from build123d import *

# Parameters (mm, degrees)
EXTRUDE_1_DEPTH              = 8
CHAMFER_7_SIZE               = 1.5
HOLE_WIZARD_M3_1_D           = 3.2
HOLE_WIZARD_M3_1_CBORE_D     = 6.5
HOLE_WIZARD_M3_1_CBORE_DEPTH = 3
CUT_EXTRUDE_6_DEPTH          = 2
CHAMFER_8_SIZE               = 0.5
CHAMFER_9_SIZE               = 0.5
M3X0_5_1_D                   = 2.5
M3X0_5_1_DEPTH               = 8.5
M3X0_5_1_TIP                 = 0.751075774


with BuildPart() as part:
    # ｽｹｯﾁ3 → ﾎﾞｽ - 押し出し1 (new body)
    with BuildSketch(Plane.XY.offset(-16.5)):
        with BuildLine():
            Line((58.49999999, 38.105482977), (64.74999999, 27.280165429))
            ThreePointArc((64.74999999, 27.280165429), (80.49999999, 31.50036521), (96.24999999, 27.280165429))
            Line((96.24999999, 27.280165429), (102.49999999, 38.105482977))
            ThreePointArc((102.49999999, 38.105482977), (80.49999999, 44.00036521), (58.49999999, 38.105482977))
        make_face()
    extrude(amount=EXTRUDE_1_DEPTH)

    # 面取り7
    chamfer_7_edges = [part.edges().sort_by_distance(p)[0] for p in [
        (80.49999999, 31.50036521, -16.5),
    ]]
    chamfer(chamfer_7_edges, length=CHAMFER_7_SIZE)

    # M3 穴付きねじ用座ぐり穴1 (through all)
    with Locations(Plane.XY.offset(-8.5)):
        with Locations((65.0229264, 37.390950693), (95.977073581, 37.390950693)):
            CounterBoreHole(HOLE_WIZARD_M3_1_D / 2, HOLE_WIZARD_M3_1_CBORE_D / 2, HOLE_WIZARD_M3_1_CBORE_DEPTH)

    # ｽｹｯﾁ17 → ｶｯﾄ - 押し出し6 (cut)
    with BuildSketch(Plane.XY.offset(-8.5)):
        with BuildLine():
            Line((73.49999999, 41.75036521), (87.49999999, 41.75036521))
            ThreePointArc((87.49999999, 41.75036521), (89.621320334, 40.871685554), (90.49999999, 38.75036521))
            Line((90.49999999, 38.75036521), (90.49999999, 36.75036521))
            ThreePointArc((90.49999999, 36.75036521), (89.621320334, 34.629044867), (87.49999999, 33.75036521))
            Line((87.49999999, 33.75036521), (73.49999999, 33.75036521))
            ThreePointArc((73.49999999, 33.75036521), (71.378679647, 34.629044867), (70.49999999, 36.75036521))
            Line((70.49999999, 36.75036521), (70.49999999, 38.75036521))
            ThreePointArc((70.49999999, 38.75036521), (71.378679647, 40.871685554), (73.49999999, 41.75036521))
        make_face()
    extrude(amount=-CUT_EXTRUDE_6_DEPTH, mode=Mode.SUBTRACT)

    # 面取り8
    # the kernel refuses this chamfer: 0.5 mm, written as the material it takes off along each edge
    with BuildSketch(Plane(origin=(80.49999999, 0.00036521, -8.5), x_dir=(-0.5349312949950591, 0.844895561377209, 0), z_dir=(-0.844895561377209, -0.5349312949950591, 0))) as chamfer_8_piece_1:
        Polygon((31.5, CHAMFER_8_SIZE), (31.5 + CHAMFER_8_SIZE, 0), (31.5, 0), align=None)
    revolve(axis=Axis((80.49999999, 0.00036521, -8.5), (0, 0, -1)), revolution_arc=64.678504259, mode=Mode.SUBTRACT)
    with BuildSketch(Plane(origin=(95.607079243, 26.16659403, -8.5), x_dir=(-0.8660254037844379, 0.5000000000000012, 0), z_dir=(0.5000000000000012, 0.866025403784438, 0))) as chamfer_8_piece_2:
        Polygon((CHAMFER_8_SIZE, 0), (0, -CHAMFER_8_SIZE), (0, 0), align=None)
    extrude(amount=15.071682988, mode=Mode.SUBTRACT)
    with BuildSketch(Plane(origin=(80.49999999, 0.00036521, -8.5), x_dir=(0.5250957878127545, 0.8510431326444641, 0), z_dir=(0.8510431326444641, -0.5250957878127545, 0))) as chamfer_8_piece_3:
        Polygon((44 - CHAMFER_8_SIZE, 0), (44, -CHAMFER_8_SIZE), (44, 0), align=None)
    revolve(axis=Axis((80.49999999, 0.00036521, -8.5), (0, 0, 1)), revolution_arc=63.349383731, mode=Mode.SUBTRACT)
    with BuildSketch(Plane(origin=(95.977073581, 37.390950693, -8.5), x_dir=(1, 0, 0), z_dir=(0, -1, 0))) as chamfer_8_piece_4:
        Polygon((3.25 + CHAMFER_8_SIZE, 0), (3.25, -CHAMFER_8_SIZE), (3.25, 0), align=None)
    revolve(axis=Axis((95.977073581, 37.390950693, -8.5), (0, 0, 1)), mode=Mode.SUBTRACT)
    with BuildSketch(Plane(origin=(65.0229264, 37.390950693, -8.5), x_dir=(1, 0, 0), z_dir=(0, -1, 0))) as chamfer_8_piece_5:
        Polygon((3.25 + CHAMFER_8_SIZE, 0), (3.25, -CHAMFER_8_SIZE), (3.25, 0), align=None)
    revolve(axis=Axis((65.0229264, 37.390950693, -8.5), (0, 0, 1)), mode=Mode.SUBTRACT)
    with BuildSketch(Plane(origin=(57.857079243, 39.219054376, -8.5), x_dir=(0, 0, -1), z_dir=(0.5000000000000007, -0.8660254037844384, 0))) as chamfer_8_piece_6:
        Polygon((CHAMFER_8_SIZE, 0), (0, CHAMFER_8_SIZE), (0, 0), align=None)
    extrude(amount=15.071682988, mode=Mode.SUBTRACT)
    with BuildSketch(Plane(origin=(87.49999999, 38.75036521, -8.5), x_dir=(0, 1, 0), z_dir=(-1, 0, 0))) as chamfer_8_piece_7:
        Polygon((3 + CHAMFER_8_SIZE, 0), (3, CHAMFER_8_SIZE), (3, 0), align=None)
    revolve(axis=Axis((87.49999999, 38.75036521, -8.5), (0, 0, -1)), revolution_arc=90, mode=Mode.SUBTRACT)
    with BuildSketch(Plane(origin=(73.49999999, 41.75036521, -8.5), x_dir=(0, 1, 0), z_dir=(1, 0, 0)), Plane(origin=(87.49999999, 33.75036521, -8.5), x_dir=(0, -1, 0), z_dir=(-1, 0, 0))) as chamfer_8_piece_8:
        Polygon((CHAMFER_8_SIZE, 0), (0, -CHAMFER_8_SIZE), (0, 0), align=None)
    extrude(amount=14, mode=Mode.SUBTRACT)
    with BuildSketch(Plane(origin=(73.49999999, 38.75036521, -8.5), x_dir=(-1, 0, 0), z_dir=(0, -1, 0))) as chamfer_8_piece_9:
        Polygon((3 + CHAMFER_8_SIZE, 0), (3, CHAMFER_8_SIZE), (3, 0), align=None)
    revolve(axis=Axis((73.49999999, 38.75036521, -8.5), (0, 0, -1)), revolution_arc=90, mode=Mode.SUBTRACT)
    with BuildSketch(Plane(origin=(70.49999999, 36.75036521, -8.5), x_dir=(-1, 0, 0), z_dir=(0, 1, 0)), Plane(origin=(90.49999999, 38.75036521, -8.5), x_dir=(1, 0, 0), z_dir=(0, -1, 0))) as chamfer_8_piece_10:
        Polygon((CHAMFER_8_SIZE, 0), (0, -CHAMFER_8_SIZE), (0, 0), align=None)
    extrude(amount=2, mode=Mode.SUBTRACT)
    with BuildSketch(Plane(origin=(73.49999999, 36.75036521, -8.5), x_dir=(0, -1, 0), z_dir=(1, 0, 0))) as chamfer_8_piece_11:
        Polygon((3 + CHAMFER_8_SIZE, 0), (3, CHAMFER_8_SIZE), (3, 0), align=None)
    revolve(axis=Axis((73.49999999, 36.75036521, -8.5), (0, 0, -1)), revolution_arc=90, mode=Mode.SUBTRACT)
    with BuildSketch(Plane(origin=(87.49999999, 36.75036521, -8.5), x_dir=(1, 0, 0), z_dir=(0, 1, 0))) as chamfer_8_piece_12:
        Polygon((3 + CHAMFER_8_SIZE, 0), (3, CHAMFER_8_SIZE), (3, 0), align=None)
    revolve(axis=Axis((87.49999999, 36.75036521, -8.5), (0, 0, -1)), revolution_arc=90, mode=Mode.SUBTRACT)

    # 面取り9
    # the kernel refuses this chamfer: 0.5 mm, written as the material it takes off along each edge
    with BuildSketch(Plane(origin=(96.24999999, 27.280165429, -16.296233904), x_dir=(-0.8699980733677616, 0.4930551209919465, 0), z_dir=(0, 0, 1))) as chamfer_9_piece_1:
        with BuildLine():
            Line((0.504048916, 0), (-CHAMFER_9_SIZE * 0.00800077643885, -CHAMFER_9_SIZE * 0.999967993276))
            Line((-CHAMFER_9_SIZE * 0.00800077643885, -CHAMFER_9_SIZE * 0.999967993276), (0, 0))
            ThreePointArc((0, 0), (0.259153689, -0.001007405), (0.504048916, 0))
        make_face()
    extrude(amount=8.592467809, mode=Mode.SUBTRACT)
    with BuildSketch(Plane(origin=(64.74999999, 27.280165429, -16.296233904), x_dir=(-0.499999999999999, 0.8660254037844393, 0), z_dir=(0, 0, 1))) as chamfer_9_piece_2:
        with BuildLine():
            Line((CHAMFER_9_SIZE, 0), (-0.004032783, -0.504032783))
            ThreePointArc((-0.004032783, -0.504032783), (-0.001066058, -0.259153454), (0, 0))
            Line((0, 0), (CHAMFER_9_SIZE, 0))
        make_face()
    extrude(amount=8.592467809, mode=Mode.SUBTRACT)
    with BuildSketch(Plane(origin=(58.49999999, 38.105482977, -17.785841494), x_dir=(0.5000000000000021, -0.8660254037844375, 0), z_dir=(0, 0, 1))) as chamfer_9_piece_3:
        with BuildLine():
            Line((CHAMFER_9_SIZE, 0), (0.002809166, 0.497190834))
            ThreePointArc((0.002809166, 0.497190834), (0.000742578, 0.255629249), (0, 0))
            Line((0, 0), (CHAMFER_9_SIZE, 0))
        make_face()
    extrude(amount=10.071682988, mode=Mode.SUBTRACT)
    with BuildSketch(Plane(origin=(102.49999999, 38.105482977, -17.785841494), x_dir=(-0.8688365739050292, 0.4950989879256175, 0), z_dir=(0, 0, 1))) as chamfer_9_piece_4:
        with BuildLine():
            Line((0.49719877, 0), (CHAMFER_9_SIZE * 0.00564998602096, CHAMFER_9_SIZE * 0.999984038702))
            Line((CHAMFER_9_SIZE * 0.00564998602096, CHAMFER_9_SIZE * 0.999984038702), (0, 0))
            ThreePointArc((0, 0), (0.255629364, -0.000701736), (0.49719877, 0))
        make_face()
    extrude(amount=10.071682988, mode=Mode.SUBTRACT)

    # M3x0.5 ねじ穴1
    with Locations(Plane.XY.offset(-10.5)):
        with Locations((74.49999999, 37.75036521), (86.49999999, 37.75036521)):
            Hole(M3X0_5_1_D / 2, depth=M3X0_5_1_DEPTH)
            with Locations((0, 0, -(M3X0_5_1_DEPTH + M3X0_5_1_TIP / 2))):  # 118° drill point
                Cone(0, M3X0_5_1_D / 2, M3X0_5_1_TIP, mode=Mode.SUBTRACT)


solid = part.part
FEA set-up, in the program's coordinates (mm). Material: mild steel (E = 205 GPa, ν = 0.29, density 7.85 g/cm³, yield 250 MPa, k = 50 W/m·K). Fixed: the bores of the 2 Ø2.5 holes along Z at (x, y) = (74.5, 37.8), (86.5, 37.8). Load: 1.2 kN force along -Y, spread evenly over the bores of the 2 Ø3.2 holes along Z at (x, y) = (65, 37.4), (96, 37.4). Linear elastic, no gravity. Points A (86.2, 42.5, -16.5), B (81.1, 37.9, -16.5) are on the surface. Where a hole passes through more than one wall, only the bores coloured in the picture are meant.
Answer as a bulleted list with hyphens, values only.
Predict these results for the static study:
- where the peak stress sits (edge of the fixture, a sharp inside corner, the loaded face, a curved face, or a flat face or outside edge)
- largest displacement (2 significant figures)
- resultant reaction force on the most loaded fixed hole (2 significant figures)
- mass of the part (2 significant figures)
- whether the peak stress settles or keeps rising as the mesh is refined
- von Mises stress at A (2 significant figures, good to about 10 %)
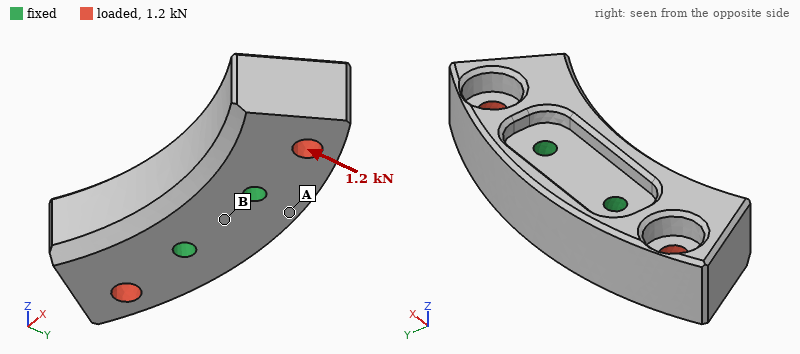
- edge of the fixture
- 4.5 µm
- 610 N
- 25 g
- keeps rising
- 19 MPa
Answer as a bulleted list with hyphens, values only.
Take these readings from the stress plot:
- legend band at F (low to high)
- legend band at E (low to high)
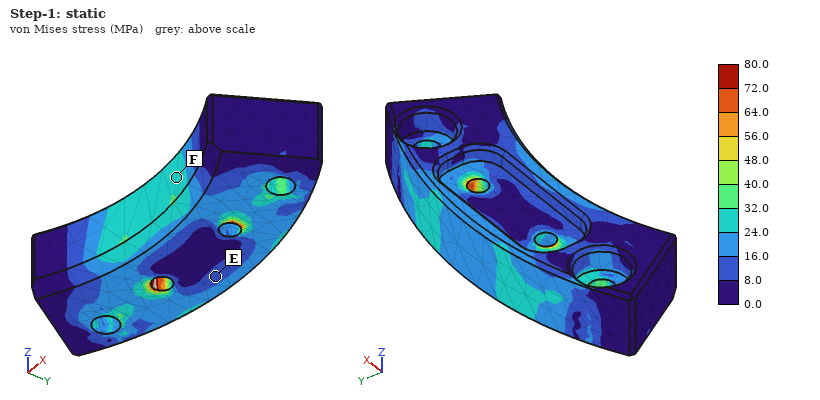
- 24.0 to 32.0 MPa
- 8.0 to 16.0 MPa
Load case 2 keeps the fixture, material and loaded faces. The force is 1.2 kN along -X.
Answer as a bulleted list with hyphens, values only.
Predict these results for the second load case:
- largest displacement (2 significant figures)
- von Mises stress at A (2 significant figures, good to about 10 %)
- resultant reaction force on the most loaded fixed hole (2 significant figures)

- 1.3 µm
- 5.4 MPa
- 600 N
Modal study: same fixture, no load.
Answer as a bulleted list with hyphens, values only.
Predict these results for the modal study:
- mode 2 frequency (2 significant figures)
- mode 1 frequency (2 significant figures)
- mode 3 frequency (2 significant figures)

- 21 kHz
- 21 kHz
- 24 kHz
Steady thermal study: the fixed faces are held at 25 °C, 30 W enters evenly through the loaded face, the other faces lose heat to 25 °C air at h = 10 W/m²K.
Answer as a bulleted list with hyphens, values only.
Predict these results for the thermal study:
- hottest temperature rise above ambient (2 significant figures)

- 53 K
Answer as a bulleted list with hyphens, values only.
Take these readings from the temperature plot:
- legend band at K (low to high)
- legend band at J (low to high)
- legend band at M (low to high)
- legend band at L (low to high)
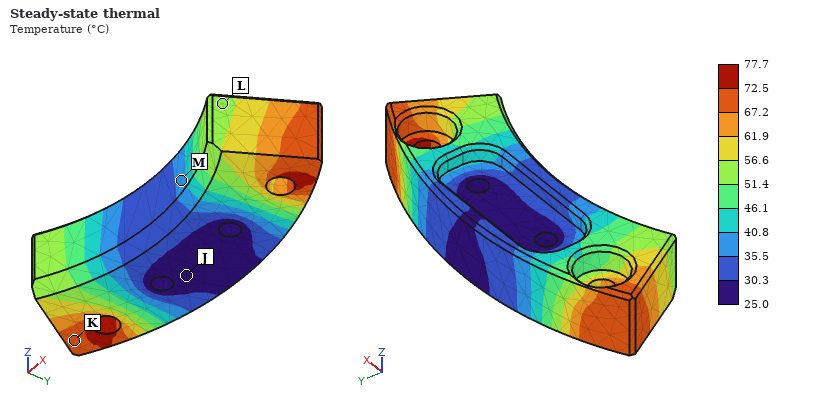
- 67.2 to 72.5 °C
- 25.0 to 30.3 °C
- 35.5 to 40.8 °C
- 51.4 to 56.6 °C
